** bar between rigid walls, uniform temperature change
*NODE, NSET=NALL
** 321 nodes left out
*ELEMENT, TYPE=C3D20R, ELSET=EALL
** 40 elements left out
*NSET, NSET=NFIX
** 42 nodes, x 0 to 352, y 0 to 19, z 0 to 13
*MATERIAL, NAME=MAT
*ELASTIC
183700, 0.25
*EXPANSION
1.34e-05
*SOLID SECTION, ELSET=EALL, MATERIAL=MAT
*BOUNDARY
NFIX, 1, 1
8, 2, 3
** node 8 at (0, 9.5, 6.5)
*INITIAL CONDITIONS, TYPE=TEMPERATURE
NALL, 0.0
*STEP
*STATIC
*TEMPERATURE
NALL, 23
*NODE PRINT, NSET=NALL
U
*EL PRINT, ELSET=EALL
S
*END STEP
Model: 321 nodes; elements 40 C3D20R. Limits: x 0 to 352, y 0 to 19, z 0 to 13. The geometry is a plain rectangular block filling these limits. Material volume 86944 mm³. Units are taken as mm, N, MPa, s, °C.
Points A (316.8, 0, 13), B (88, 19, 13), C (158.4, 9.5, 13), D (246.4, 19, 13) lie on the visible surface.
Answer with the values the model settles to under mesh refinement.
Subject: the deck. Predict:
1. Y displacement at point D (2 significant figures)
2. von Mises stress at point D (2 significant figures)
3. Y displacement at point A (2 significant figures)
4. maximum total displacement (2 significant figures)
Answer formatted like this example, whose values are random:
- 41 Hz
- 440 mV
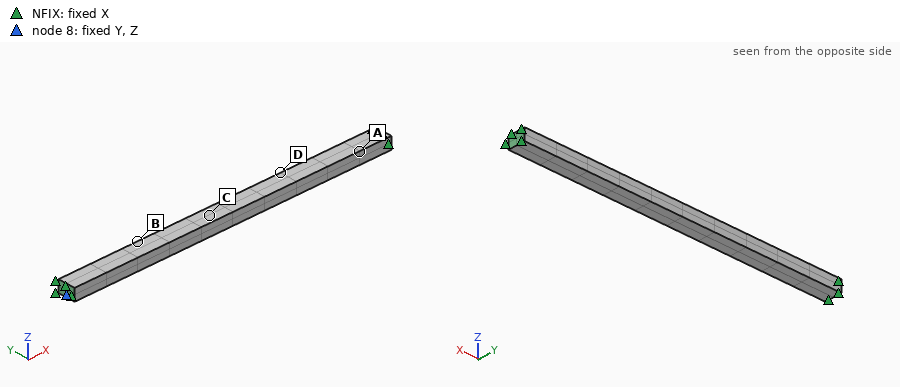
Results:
- 0.0034 mm
- 57 MPa
- -0.0039 mm
- 0.0045 mm
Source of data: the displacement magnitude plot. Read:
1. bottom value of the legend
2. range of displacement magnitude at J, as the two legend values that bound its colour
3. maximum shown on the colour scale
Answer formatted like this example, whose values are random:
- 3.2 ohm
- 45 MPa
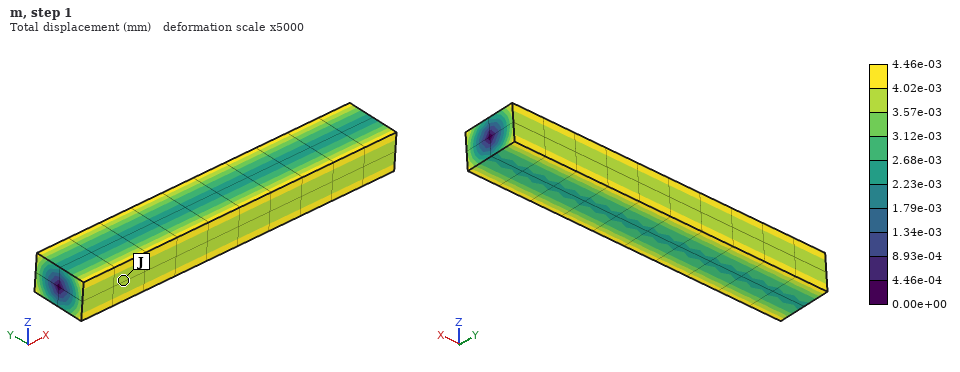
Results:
- 0.00e+00 mm
- 3.57e-03 to 4.02e-03 mm
- 4.46e-03 mm
